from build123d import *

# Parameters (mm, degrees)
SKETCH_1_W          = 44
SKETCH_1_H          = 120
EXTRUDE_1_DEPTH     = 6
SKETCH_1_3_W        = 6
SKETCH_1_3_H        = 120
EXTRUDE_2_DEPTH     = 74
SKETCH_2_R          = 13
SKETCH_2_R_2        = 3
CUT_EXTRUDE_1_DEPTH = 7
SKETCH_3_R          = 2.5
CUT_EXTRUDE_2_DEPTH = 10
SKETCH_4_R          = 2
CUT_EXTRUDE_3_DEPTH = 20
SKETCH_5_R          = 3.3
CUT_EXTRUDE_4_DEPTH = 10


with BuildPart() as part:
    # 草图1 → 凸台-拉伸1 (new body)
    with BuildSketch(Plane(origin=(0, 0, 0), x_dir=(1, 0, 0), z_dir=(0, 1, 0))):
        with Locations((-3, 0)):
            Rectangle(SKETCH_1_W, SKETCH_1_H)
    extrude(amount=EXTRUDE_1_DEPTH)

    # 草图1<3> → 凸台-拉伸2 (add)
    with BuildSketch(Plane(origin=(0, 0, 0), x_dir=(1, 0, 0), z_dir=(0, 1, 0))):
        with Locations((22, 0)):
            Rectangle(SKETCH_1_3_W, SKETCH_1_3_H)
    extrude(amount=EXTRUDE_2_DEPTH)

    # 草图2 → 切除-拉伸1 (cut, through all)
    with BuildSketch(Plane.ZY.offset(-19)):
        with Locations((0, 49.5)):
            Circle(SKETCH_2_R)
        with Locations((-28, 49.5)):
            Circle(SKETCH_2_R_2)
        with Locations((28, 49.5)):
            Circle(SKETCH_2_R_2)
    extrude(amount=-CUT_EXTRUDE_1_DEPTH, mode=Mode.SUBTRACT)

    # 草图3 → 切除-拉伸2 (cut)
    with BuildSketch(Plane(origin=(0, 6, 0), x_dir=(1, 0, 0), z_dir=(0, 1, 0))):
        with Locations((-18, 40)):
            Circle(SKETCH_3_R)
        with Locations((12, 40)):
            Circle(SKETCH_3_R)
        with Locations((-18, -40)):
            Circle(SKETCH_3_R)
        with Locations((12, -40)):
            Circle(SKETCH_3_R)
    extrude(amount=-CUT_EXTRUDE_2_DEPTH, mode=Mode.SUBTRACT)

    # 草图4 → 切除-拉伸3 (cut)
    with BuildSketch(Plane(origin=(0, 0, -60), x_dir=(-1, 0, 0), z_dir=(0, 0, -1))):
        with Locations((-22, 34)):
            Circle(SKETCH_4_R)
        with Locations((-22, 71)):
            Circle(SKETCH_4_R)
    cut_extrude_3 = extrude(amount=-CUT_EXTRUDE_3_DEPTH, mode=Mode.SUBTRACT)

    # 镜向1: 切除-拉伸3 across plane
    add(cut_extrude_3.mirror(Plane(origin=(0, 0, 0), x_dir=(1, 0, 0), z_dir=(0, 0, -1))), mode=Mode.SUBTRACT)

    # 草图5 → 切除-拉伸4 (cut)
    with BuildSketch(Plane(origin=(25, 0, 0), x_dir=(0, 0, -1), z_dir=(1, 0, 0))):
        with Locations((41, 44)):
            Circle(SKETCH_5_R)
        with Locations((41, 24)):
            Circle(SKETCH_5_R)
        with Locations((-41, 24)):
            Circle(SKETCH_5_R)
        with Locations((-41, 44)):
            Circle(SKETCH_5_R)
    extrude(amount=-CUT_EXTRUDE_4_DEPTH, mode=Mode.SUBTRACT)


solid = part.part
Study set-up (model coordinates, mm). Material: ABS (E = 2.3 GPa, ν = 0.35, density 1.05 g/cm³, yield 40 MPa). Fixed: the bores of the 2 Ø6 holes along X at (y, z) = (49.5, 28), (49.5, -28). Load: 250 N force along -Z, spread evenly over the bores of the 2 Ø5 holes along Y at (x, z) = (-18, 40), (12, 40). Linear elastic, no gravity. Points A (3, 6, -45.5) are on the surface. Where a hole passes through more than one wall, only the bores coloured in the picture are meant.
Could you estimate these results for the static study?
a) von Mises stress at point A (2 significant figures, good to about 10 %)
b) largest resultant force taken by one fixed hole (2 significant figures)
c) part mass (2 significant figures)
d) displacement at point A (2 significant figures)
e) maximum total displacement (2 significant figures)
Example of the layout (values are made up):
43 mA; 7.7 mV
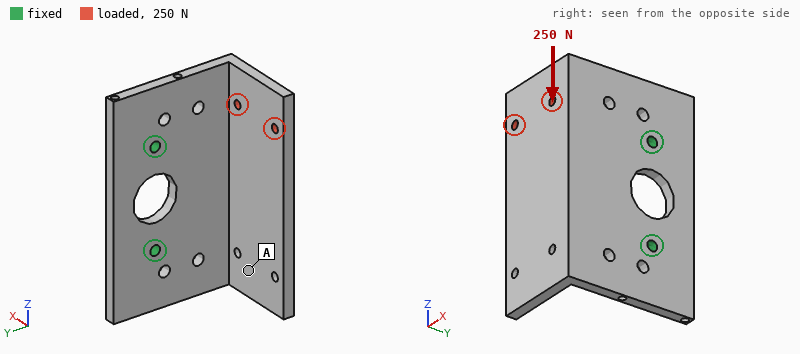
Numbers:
2.5 MPa; 240 N; 83 g; 0.91 mm; 1.5 mm
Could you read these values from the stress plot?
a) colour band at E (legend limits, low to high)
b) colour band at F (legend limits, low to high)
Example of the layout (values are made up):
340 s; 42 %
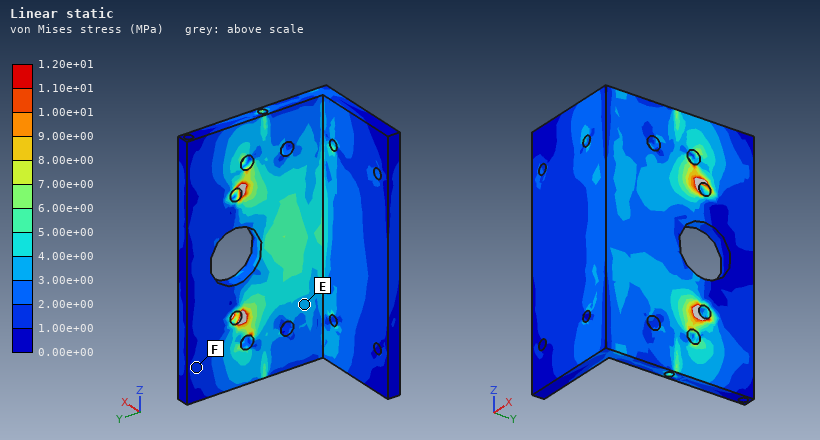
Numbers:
3.00e+00 to 4.00e+00 MPa; 1.00e+00 to 2.00e+00 MPa
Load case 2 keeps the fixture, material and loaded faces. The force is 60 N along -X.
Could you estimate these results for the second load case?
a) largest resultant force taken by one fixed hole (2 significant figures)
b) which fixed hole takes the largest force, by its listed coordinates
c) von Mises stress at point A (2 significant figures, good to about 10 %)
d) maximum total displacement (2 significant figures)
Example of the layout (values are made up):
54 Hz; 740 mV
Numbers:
63 N; (49.5, 28); 0.88 MPa; 1.5 mm
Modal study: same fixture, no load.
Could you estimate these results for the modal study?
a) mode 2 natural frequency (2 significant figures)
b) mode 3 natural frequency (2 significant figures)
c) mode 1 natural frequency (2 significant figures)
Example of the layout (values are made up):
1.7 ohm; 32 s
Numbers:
310 Hz; 580 Hz; 190 Hz
